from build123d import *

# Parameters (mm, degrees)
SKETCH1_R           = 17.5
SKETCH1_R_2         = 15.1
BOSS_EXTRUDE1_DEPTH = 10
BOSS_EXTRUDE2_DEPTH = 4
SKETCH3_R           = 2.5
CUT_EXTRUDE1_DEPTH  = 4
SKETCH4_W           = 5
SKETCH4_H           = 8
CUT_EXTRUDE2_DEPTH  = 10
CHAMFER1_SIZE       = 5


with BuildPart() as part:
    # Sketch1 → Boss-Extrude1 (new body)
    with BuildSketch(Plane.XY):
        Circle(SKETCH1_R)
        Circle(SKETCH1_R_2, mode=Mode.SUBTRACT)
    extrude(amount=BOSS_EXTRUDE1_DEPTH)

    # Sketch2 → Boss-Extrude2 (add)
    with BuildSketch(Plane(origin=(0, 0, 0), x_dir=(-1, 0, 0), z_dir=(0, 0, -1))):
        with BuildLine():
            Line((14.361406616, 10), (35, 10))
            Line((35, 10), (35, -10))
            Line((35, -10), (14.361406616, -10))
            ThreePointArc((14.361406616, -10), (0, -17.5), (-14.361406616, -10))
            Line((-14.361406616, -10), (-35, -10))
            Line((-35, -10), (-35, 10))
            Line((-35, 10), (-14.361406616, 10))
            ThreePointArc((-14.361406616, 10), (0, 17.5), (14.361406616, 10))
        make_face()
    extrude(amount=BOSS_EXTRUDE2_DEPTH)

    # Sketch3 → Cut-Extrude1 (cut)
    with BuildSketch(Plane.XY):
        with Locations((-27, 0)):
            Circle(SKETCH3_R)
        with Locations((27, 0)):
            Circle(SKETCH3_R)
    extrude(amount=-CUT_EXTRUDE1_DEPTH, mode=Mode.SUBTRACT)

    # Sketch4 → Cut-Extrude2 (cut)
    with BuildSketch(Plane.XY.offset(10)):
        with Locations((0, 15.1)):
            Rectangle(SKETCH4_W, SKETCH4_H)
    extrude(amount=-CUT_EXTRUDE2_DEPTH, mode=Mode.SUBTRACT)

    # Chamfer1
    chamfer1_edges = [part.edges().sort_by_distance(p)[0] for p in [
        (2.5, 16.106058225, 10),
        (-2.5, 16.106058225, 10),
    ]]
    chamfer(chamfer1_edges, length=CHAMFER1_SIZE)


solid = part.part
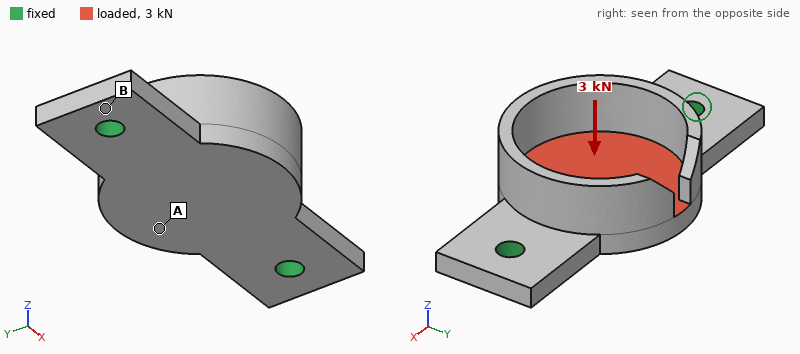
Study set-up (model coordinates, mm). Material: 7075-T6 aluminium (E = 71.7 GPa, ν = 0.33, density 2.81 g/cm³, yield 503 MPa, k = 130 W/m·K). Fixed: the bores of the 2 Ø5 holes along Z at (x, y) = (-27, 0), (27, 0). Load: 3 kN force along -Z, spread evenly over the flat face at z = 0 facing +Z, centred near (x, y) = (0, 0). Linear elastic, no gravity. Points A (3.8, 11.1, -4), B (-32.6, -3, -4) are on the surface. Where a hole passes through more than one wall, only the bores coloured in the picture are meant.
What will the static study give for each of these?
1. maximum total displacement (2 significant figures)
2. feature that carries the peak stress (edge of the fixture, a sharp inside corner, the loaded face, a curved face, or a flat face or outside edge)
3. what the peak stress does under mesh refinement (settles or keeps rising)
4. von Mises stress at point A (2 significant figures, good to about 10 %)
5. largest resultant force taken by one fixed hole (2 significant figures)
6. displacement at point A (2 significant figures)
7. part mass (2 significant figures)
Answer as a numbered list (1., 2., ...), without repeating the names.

1. 0.22 mm
2. edge of the fixture
3. keeps rising
4. 120 MPa
5. 1.5 kN
6. 0.18 mm
7. 25 g
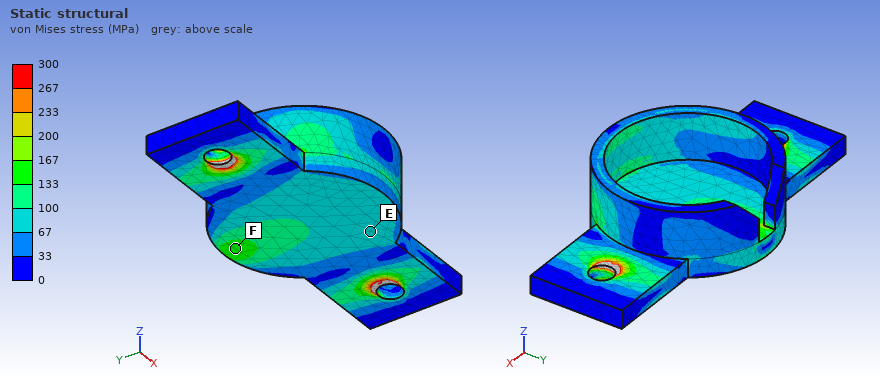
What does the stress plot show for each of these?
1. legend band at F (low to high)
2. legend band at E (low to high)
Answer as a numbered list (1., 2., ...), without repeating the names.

1. 133 to 167 MPa
2. 67 to 100 MPa
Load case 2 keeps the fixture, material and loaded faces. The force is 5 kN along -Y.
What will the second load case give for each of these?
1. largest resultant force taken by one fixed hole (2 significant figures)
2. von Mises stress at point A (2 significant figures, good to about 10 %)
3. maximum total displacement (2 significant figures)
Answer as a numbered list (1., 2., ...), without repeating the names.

1. 2.5 kN
2. 43 MPa
3. 0.12 mm
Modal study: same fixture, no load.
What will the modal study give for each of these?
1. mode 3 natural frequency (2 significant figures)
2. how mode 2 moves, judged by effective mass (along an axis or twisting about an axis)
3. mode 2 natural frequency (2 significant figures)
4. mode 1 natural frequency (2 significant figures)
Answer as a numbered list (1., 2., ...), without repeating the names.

1. 14 kHz
2. along Z
3. 5700 Hz
4. 5100 Hz
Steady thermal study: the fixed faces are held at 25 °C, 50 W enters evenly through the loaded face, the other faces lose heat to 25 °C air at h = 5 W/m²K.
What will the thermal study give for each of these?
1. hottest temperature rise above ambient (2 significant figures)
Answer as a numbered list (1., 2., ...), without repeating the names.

1. 43 K
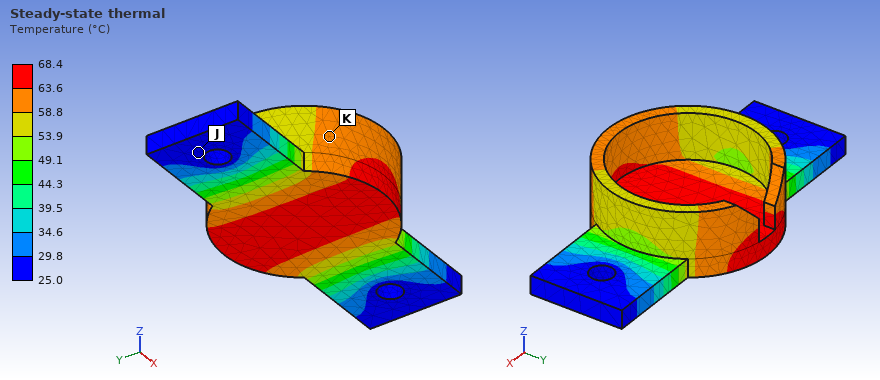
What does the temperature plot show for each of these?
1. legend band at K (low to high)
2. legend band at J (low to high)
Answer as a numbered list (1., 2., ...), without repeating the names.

1. 58.8 to 63.6 °C
2. 25.0 to 29.8 °C
